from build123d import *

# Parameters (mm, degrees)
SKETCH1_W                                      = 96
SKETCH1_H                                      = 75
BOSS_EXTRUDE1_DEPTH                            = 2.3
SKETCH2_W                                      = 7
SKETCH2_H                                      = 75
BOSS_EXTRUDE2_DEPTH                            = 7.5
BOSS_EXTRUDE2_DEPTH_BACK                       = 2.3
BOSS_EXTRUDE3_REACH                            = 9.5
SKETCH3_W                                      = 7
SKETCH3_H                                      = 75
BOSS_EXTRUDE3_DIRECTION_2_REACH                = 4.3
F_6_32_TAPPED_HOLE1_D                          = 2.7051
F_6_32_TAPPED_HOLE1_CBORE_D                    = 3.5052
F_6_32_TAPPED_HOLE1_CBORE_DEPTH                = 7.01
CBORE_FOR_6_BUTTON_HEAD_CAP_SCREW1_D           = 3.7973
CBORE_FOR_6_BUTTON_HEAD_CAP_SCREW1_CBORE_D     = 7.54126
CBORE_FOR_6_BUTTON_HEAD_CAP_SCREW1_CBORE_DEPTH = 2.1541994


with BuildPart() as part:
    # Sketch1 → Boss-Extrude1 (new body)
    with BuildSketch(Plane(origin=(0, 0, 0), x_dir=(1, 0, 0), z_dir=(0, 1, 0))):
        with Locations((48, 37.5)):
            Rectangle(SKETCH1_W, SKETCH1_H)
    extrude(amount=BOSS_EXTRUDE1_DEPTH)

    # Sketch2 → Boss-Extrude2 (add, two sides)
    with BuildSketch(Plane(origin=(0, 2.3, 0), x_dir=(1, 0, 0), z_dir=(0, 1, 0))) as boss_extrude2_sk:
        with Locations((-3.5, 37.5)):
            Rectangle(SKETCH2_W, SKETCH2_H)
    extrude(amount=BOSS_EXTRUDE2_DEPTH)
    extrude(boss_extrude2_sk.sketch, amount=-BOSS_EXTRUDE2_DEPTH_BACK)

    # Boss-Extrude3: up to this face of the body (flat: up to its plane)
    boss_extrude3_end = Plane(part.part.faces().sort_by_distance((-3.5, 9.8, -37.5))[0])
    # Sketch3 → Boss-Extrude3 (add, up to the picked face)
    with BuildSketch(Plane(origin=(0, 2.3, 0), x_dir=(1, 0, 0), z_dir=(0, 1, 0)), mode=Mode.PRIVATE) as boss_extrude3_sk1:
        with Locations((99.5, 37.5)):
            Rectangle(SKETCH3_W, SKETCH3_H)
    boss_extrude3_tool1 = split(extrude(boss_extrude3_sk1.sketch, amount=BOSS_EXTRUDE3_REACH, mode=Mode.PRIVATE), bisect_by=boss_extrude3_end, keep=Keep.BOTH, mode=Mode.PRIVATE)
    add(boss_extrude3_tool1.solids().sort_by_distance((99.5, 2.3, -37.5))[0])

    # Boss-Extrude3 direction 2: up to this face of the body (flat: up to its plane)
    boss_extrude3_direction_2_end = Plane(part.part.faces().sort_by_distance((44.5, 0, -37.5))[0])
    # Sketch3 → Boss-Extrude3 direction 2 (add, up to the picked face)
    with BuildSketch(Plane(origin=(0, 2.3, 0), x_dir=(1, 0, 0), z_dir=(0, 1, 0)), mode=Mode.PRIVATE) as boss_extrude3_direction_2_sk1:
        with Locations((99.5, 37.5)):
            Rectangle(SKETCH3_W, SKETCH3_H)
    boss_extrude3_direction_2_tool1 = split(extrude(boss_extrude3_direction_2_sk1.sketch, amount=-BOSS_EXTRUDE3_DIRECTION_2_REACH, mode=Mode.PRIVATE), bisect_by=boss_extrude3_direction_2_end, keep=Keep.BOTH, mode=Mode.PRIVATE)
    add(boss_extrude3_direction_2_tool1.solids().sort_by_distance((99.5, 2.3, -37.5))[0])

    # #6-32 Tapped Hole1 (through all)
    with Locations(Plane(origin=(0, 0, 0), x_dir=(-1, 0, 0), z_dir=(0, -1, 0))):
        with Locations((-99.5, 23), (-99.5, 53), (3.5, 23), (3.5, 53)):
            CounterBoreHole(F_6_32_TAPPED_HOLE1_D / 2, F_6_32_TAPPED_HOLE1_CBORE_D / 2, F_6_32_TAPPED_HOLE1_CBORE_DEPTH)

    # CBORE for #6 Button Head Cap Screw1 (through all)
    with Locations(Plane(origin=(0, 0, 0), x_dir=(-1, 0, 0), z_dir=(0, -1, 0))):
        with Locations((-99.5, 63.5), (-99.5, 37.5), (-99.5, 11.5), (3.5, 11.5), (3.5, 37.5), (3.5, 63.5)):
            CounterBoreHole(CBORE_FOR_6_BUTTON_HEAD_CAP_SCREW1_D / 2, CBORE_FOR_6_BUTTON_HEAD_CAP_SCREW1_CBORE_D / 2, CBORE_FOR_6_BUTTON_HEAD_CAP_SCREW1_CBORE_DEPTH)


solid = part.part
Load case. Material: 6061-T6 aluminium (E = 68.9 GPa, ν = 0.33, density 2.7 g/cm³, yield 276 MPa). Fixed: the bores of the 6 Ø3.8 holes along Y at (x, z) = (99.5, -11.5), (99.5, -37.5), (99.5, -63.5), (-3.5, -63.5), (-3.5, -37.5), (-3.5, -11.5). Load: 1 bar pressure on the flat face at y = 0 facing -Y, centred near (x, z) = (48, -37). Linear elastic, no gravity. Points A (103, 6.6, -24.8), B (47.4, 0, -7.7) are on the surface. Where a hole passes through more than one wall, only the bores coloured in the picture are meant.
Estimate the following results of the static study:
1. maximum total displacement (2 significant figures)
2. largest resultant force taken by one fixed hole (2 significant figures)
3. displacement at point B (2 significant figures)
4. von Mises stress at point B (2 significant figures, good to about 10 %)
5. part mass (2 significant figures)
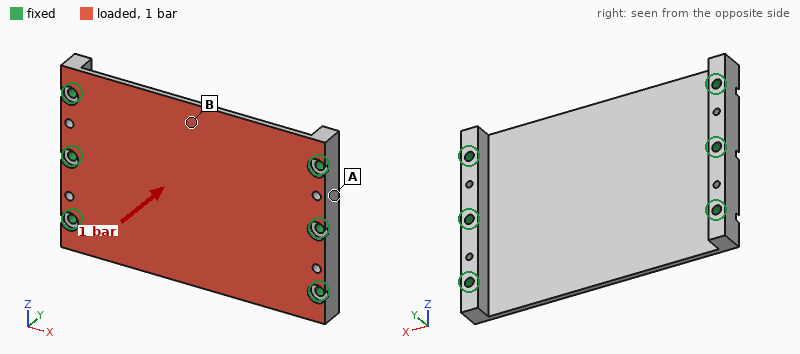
0.38 mm
240 N
0.36 mm
49 MPa
69 g
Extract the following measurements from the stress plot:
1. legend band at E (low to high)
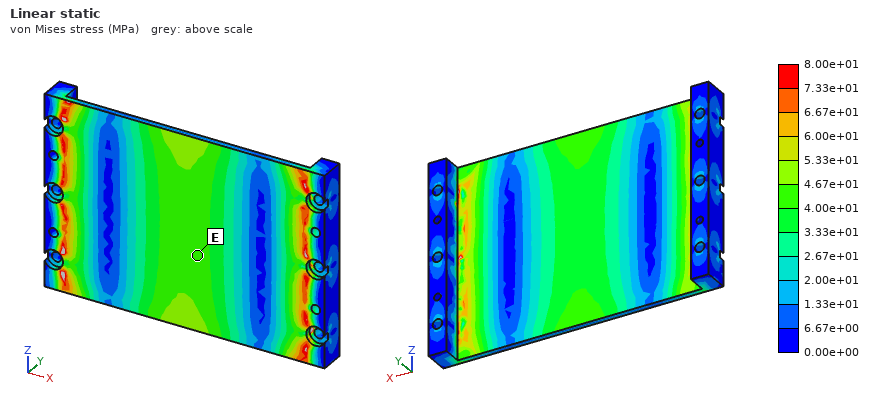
4.00e+01 to 4.67e+01 MPa
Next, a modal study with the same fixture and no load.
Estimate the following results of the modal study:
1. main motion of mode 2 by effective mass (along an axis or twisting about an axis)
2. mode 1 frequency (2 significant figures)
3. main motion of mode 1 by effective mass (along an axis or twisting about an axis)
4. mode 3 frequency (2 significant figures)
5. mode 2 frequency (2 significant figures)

twisting about X
1200 Hz
along Y
3300 Hz
1600 Hz
